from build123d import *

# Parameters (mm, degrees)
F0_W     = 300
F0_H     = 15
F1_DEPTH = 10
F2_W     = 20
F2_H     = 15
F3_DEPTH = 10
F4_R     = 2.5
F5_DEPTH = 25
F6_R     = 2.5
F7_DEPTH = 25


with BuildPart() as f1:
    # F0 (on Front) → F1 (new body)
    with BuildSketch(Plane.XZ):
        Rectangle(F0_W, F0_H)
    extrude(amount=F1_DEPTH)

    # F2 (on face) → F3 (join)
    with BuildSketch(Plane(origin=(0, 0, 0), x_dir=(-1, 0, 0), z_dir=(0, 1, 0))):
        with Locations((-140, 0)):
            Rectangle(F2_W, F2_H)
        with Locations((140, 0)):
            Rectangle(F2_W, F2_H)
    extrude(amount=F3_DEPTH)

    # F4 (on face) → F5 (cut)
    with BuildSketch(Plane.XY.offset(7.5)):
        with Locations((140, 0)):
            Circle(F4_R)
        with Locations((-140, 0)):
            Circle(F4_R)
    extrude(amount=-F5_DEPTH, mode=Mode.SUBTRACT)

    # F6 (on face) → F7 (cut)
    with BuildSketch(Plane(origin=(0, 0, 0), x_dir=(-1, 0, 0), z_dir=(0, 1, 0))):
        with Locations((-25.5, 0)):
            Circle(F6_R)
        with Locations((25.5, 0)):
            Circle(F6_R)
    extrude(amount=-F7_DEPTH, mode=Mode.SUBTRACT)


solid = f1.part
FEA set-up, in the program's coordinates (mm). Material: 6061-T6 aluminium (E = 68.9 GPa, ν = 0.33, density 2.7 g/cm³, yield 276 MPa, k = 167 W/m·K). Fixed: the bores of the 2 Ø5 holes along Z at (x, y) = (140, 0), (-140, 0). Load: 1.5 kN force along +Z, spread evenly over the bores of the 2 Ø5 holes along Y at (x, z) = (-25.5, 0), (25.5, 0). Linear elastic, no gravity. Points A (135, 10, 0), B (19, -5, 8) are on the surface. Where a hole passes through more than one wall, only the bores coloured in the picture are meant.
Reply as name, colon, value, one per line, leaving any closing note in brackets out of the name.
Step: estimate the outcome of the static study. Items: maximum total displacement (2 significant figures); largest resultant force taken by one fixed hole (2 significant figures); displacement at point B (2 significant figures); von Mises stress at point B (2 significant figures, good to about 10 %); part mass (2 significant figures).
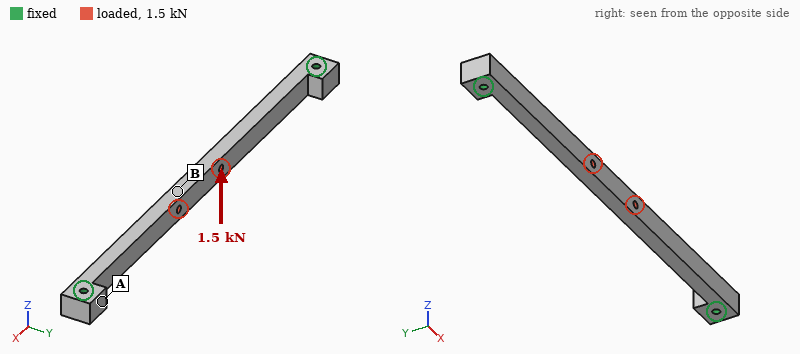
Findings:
maximum total displacement: 0.82 mm
largest resultant force taken by one fixed hole: 750 N
displacement at point B: 0.78 mm
von Mises stress at point B: 96 MPa
part mass: 140 g
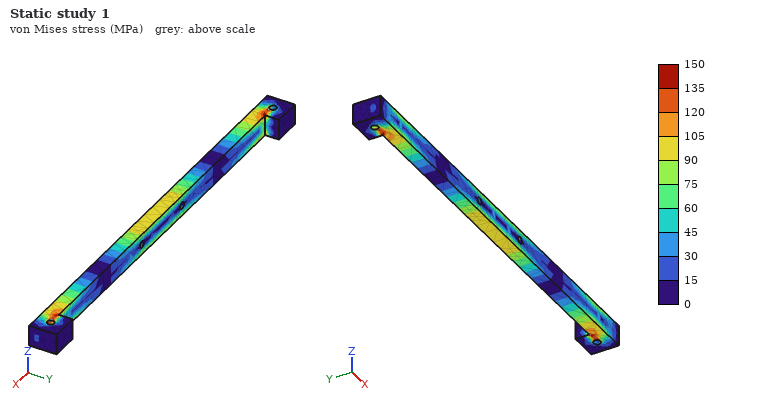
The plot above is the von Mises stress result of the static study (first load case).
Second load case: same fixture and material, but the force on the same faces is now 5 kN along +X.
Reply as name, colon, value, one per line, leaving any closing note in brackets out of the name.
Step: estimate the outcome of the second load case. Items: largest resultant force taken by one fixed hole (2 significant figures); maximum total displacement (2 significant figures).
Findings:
largest resultant force taken by one fixed hole: 2.5 kN
maximum total displacement: 33 µm
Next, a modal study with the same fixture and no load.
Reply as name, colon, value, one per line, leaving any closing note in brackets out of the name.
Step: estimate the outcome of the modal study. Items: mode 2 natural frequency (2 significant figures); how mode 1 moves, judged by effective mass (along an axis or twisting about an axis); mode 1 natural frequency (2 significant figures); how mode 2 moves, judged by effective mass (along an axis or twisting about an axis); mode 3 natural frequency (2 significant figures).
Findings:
mode 2 natural frequency: 1000 Hz
how mode 1 moves, judged by effective mass: along Y
mode 1 natural frequency: 680 Hz
how mode 2 moves, judged by effective mass: along Z
mode 3 natural frequency: 1800 Hz
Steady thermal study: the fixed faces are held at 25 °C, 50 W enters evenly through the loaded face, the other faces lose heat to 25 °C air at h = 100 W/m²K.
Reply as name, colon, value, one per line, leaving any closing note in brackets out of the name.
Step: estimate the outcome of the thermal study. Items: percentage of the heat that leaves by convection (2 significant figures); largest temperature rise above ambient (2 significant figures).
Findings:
percentage of the heat that leaves by convection: 70 %
largest temperature rise above ambient: 51 K
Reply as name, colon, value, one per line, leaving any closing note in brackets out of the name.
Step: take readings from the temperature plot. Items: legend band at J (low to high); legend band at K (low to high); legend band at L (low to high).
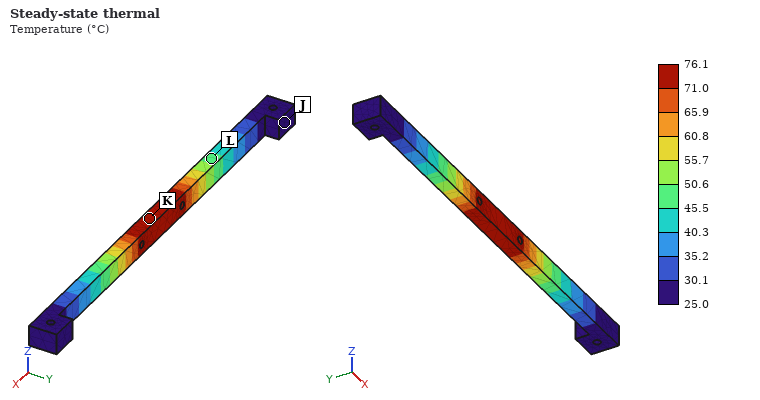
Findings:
legend band at J: 25.0 to 30.1 °C
legend band at K: 71.0 to 76.1 °C
legend band at L: 45.5 to 50.6 °C
